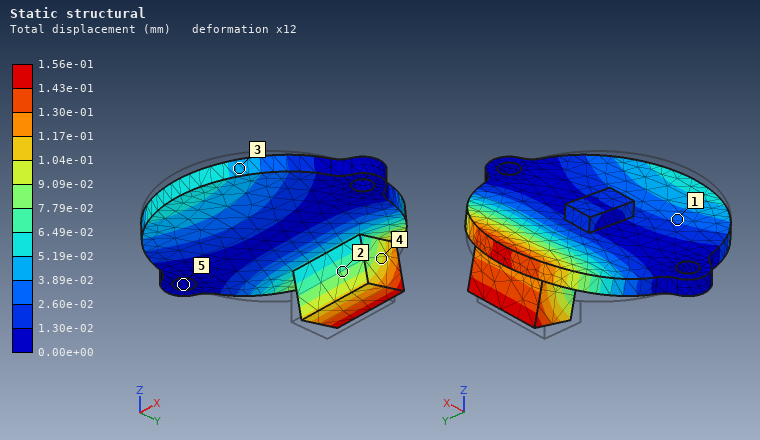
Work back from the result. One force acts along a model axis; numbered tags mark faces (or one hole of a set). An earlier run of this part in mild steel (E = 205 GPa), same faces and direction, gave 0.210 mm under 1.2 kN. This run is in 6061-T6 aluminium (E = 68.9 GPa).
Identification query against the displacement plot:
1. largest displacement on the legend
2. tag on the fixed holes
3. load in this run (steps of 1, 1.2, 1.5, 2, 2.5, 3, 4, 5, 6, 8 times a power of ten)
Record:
1.56e-01 mm
5
300 N
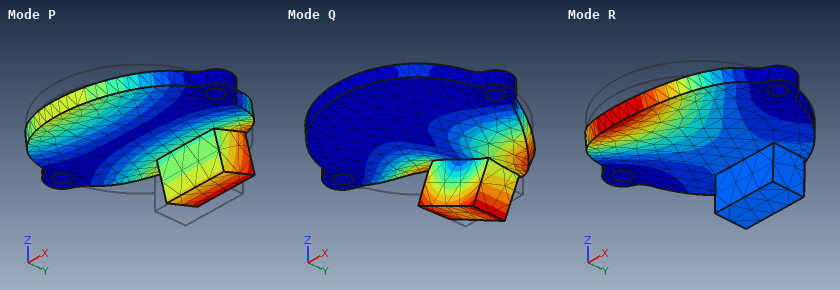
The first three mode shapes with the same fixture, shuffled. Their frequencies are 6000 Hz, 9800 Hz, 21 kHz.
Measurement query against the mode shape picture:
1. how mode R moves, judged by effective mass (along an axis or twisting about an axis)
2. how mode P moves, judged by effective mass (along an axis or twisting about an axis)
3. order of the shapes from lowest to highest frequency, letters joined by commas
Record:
along Z
along Z
P, R, Q
